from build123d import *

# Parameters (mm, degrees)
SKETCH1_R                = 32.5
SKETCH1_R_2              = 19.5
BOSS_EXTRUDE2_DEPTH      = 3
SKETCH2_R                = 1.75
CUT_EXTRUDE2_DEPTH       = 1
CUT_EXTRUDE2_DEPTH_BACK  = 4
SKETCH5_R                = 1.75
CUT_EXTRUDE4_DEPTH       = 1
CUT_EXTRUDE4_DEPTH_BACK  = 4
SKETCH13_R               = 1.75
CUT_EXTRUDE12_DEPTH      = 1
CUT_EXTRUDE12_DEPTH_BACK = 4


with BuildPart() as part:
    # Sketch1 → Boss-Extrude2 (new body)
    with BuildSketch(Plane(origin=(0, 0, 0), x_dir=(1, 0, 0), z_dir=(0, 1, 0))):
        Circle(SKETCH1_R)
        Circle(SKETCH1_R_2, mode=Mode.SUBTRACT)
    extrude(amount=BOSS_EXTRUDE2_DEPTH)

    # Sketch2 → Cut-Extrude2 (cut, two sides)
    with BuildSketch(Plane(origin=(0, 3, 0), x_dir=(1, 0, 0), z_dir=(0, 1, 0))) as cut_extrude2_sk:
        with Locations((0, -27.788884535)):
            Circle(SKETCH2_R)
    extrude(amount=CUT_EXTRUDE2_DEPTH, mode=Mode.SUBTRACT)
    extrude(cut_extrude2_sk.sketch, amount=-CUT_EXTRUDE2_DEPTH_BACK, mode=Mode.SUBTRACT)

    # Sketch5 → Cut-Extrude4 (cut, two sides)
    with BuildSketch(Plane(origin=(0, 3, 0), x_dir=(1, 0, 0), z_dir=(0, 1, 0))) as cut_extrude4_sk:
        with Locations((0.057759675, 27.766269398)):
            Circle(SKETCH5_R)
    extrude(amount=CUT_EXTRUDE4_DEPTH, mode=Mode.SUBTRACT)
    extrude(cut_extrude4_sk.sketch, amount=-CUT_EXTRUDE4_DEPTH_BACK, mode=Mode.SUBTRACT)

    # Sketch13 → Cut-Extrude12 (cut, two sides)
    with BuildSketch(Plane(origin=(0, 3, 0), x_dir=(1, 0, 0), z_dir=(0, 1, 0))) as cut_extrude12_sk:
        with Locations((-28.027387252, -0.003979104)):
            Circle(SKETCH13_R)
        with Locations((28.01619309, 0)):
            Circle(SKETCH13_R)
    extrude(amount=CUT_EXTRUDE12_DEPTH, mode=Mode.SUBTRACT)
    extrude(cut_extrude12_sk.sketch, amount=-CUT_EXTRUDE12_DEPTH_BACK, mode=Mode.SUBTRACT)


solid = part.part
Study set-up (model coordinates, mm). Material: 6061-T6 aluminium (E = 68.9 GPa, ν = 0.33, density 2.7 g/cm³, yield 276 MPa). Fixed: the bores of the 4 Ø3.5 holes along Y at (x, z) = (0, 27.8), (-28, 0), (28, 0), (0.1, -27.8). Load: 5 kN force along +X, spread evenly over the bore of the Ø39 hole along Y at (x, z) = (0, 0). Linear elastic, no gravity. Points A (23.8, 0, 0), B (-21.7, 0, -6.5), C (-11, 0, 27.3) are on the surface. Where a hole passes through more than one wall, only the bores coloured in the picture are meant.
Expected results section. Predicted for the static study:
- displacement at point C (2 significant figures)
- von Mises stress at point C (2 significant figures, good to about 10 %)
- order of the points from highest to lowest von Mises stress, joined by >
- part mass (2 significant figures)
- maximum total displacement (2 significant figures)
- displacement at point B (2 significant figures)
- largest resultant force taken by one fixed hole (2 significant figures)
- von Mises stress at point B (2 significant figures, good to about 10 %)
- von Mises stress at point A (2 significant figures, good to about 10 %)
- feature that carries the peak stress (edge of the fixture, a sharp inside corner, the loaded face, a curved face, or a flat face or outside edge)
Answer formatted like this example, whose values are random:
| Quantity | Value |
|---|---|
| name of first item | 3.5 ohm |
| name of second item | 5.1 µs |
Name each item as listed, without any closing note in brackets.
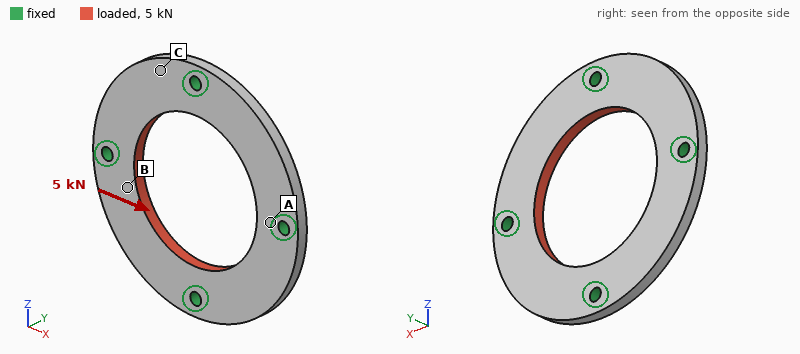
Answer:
| Quantity | Value |
|---|---|
| displacement at point C | 5.4 µm |
| von Mises stress at point C | 19 MPa |
| order of the points from highest to lowest von Mises stress, joined by > | A > B > C |
| part mass | 17 g |
| maximum total displacement | 11 µm |
| displacement at point B | 5.6 µm |
| largest resultant force taken by one fixed hole | 1.5 kN |
| von Mises stress at point B | 28 MPa |
| von Mises stress at point A | 38 MPa |
| feature that carries the peak stress | edge of the fixture |
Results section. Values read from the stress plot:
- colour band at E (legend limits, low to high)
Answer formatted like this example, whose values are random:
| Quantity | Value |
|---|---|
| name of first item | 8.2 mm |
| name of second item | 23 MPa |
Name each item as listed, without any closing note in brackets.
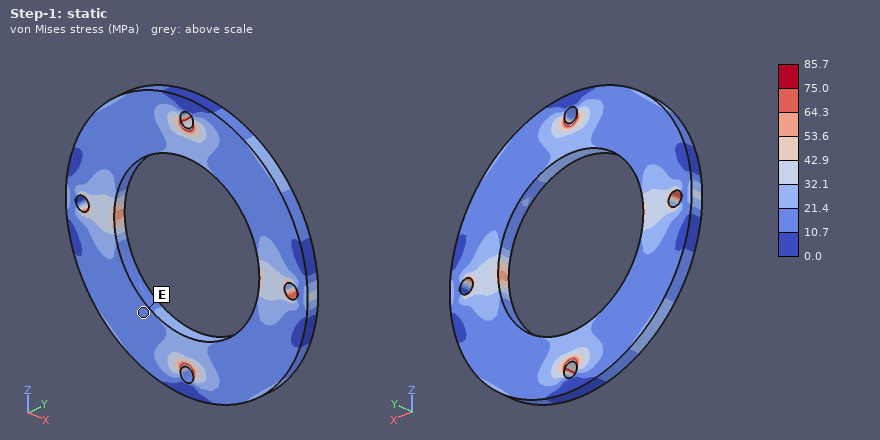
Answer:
| Quantity | Value |
|---|---|
| colour band at E | 10.7 to 21.4 MPa |
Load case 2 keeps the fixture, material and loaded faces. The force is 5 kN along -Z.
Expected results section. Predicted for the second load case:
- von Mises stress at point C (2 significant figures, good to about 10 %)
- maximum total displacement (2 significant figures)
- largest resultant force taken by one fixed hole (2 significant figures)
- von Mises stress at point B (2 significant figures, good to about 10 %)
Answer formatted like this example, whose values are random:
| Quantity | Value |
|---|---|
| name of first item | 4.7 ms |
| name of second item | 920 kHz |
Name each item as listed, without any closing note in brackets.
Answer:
| Quantity | Value |
|---|---|
| von Mises stress at point C | 12 MPa |
| maximum total displacement | 11 µm |
| largest resultant force taken by one fixed hole | 1.5 kN |
| von Mises stress at point B | 20 MPa |
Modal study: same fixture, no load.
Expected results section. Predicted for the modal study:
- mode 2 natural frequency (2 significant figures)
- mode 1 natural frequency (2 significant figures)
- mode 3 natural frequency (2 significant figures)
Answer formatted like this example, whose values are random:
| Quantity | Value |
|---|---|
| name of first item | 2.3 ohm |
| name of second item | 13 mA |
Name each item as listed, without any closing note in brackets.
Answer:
| Quantity | Value |
|---|---|
| mode 2 natural frequency | 8200 Hz |
| mode 1 natural frequency | 7800 Hz |
| mode 3 natural frequency | 8200 Hz |
